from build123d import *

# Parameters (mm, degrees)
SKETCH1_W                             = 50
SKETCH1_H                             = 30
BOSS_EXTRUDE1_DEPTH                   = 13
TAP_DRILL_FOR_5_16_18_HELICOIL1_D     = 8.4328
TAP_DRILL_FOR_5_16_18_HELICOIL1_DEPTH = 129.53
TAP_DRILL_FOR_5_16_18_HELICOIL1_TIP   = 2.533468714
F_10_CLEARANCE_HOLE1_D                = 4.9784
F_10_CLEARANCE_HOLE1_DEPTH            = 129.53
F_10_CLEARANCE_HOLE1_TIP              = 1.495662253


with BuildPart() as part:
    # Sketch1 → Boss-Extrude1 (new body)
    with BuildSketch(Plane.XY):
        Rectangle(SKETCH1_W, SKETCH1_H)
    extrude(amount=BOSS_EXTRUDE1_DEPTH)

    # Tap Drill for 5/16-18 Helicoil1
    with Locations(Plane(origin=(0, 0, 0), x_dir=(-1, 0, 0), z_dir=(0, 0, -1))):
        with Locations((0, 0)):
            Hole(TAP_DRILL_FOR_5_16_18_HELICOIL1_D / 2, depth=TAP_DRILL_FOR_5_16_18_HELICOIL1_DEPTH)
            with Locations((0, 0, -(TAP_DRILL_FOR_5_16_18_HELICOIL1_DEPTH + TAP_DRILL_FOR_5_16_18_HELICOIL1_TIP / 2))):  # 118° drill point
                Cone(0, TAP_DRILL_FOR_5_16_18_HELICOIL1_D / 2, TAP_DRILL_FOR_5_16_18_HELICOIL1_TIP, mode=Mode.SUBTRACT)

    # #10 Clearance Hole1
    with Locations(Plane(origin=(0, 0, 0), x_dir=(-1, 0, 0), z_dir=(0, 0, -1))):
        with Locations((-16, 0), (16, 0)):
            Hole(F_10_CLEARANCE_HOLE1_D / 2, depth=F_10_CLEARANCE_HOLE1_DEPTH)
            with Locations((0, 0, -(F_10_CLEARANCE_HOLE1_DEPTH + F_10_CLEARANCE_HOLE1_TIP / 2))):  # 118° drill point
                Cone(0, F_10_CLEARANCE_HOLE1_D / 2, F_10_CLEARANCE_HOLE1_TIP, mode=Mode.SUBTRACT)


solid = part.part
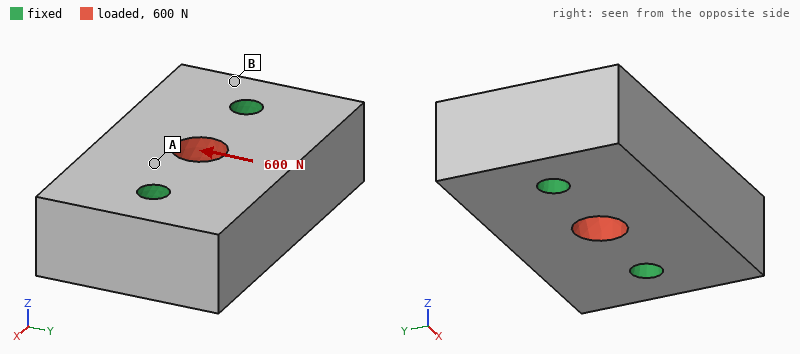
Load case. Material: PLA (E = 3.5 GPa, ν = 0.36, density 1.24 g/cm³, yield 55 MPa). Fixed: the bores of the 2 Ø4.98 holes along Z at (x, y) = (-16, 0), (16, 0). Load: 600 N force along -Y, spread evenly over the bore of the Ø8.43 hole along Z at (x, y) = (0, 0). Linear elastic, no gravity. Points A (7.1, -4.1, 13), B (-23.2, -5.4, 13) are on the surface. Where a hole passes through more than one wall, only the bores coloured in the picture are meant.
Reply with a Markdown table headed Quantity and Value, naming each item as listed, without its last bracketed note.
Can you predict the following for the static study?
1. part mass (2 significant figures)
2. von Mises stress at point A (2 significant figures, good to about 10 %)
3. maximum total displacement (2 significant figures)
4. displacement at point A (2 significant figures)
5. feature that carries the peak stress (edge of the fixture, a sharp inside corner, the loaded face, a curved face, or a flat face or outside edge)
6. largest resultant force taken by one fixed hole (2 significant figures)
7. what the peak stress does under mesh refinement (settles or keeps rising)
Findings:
| Quantity | Value |
|---|---|
| part mass | 23 g |
| von Mises stress at point A | 1.7 MPa |
| maximum total displacement | 14 µm |
| displacement at point A | 8.7 µm |
| feature that carries the peak stress | edge of the fixture |
| largest resultant force taken by one fixed hole | 300 N |
| what the peak stress does under mesh refinement | keeps rising |
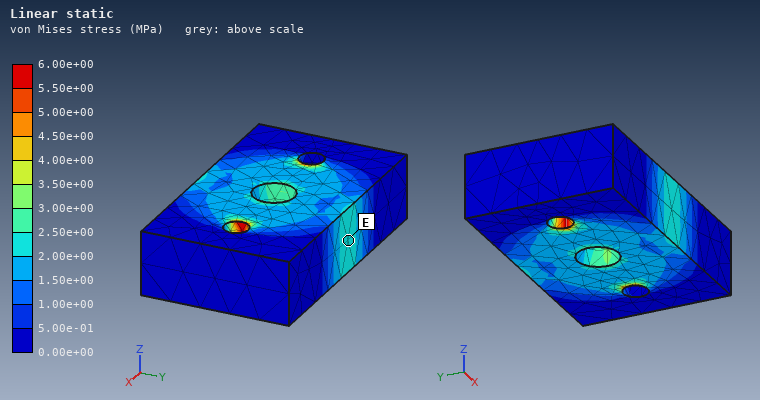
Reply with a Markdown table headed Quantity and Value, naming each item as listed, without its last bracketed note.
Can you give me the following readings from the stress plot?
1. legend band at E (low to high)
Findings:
| Quantity | Value |
|---|---|
| legend band at E | 2.00e+00 to 2.50e+00 MPa |
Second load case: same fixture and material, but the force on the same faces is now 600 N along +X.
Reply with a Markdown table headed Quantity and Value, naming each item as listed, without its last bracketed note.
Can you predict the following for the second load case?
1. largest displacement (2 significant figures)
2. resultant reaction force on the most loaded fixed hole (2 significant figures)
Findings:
| Quantity | Value |
|---|---|
| largest displacement | 7.0 µm |
| resultant reaction force on the most loaded fixed hole | 300 N |
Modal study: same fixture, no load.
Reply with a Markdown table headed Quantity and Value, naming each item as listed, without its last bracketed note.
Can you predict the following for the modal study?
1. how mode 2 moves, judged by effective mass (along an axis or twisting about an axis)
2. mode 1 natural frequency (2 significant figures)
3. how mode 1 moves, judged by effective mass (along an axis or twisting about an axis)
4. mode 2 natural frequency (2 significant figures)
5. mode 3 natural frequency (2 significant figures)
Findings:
| Quantity | Value |
|---|---|
| how mode 2 moves, judged by effective mass | along Z |
| mode 1 natural frequency | 7900 Hz |
| how mode 1 moves, judged by effective mass | twisting about X |
| mode 2 natural frequency | 9200 Hz |
| mode 3 natural frequency | 11 kHz |
